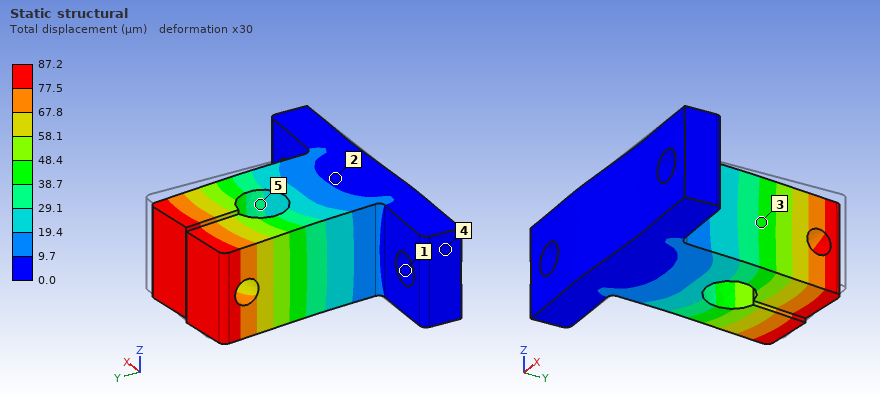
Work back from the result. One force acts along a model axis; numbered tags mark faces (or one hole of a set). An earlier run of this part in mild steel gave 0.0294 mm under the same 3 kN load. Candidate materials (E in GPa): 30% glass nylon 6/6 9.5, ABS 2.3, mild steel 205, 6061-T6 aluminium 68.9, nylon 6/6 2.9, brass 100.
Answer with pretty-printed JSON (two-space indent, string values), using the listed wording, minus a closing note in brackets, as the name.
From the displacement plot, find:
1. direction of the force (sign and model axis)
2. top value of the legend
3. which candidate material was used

{
  "direction of the force": "-X",
  "top value of the legend": "87.2 µm",
  "which candidate material was used": "6061-T6 aluminium"
}
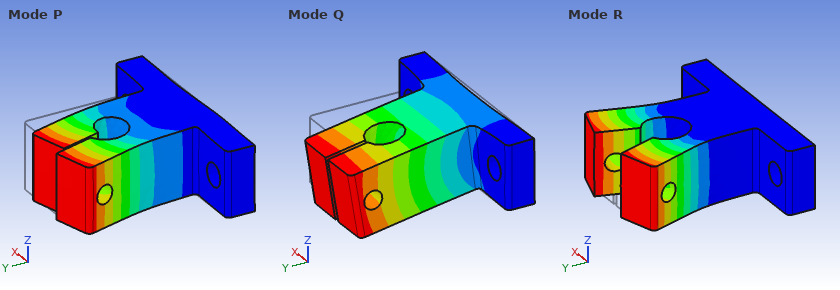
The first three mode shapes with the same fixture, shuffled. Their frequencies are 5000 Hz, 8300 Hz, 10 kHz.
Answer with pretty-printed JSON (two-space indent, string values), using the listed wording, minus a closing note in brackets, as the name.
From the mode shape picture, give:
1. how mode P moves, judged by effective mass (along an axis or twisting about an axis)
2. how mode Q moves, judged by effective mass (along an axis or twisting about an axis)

{
  "how mode P moves, judged by effective mass": "along X",
  "how mode Q moves, judged by effective mass": "along Z"
}
